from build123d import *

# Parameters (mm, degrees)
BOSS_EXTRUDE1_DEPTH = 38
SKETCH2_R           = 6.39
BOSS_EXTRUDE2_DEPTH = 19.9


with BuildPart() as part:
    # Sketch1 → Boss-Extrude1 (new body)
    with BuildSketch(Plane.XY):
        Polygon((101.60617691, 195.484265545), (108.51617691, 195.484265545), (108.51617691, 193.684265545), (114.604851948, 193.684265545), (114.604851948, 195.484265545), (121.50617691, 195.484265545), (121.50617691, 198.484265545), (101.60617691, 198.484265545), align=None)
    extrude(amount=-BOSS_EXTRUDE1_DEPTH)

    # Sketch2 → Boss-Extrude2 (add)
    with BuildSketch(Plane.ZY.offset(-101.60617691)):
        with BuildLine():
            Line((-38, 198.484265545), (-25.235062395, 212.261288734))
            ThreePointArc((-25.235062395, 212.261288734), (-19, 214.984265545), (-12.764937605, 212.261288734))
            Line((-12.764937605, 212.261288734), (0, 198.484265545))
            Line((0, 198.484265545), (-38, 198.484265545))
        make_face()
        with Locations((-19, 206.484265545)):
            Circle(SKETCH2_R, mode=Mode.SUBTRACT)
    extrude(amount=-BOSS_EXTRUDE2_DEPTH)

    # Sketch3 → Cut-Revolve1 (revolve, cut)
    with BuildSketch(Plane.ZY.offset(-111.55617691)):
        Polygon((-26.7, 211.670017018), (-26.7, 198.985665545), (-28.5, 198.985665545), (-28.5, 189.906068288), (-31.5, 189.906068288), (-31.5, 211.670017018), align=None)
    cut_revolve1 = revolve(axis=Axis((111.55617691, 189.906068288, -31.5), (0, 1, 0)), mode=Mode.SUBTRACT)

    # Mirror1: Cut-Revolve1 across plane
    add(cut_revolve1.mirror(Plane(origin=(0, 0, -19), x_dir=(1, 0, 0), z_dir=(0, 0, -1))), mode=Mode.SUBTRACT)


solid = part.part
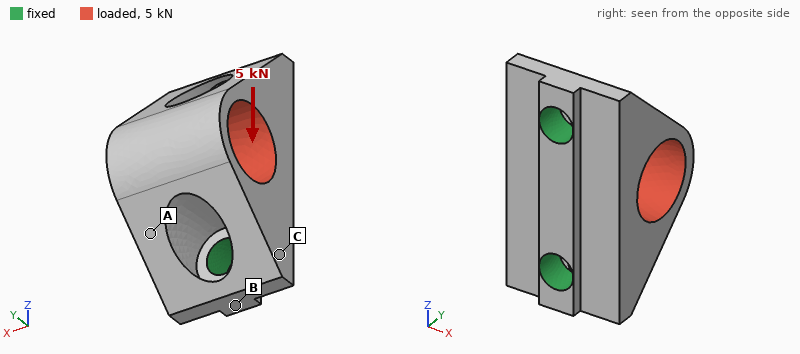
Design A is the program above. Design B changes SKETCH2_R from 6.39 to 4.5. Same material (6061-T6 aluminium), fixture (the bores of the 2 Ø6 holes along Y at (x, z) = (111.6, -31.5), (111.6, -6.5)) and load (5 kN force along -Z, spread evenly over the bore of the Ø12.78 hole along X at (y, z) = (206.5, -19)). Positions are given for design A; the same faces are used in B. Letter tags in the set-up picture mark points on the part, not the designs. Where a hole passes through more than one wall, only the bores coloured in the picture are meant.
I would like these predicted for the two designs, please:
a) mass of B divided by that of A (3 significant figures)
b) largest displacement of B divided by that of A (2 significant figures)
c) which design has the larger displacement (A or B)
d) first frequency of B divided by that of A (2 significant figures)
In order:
1.21
0.49
A
0.87
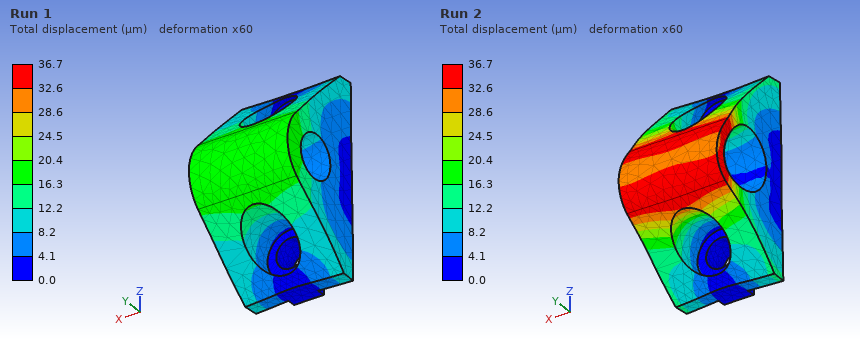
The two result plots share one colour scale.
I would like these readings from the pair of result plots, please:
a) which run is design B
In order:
Run 1
